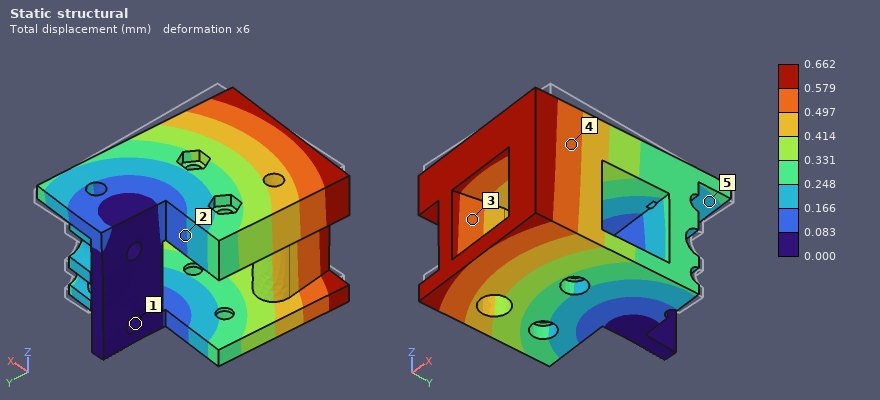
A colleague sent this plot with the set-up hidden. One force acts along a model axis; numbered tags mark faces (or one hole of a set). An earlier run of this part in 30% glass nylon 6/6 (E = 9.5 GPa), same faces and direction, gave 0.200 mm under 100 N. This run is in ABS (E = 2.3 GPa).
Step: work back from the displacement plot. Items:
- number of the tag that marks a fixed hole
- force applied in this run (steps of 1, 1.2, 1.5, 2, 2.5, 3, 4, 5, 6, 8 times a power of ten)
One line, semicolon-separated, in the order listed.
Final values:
1; 80 N
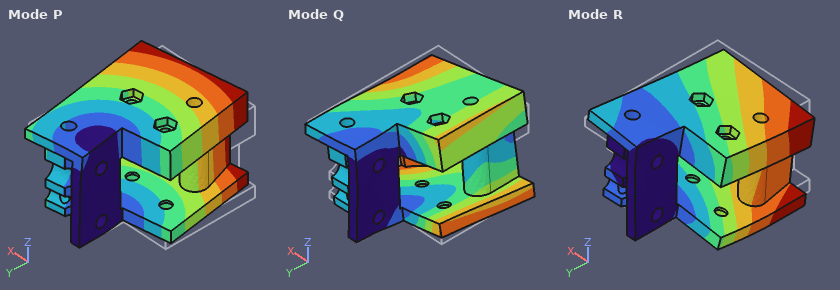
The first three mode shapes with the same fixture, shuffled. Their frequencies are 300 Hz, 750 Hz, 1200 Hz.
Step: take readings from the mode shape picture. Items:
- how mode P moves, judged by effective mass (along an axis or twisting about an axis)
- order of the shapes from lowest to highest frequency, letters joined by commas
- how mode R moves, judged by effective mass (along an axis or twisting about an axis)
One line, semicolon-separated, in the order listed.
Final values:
along X; P, R, Q; along Z
